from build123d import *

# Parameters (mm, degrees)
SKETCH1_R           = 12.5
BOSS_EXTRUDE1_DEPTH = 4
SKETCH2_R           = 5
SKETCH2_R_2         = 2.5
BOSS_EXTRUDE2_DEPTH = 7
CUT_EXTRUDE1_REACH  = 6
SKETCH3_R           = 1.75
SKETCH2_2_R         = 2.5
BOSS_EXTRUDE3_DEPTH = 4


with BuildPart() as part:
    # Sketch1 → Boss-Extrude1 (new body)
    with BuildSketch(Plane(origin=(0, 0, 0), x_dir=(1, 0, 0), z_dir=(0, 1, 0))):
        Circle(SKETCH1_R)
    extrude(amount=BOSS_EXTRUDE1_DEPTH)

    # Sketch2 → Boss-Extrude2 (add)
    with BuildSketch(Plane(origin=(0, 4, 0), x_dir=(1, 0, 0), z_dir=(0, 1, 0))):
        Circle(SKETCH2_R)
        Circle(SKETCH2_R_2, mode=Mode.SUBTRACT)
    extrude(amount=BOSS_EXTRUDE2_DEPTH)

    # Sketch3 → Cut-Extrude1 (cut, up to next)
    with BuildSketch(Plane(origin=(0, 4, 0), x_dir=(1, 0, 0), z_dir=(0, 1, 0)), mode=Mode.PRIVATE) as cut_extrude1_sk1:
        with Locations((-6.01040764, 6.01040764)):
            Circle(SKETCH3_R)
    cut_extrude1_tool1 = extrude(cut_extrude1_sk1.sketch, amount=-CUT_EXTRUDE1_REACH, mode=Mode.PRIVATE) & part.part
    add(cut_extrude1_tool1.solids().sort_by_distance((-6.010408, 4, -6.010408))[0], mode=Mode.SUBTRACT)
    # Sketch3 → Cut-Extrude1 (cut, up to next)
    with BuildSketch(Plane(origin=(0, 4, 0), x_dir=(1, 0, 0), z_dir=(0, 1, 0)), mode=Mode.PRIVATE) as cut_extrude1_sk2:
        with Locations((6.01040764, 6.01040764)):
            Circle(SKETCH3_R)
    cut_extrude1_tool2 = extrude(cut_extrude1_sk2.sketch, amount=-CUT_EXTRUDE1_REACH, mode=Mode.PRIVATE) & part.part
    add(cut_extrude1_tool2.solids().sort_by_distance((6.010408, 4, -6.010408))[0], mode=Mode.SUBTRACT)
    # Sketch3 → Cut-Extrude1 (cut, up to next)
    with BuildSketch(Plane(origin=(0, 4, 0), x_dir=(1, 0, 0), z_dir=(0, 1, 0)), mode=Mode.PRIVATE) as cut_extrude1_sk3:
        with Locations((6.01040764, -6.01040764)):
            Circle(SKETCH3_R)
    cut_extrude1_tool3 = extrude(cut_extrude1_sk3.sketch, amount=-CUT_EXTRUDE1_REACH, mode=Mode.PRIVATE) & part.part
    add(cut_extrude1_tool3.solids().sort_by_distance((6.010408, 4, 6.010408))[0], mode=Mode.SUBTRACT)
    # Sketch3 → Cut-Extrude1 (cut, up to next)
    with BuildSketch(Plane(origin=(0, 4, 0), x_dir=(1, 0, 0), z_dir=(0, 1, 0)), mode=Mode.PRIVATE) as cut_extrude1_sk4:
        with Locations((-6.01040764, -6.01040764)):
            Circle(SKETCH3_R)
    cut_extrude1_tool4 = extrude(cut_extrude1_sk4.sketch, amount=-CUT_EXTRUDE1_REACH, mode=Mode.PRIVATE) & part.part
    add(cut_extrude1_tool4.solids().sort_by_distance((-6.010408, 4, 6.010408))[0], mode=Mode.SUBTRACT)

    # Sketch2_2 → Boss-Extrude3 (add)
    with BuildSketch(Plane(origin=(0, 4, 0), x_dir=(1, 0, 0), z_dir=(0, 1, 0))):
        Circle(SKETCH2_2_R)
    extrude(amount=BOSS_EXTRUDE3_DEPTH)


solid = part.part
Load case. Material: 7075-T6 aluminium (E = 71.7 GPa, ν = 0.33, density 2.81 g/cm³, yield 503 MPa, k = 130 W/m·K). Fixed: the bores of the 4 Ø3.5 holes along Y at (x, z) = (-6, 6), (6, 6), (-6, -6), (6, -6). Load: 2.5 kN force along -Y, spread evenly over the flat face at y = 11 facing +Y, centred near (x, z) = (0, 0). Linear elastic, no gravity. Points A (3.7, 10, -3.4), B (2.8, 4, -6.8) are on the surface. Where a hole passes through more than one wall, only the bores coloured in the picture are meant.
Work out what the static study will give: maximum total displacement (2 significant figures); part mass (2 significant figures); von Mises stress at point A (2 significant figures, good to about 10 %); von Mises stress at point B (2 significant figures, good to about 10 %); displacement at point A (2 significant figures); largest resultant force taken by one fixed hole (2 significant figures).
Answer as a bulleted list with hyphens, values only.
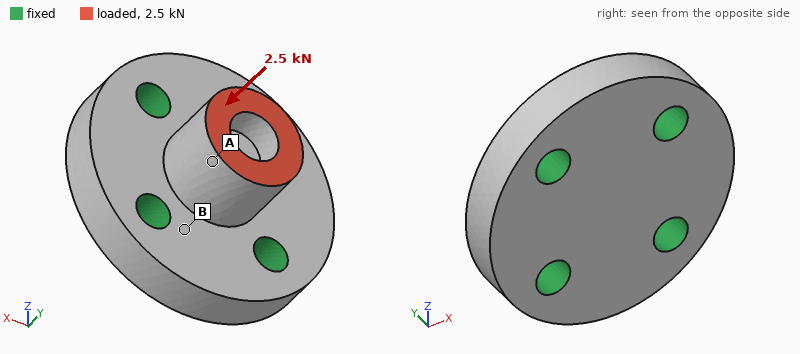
- 8.2 µm
- 6.5 g
- 43 MPa
- 13 MPa
- 7.5 µm
- 650 N
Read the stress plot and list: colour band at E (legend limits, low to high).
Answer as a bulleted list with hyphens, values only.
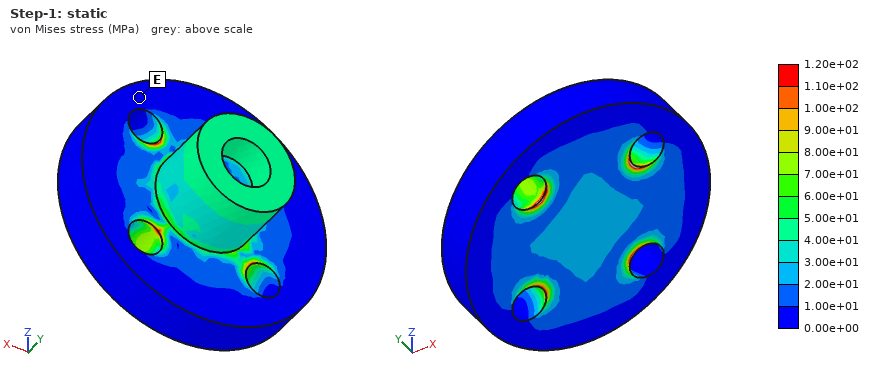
- 0.00e+00 to 1.00e+01 MPa
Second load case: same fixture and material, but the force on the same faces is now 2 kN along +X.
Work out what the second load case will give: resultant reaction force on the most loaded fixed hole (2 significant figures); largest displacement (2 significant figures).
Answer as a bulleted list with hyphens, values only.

- 990 N
- 37 µm
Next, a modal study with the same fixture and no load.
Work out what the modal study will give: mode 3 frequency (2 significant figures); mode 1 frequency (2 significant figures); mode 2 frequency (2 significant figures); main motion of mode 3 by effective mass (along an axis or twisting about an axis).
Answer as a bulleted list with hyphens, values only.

- 73 kHz
- 57 kHz
- 57 kHz
- along Y
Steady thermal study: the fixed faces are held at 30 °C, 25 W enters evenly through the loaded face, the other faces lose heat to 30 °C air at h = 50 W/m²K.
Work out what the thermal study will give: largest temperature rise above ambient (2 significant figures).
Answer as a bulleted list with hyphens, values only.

- 28 K
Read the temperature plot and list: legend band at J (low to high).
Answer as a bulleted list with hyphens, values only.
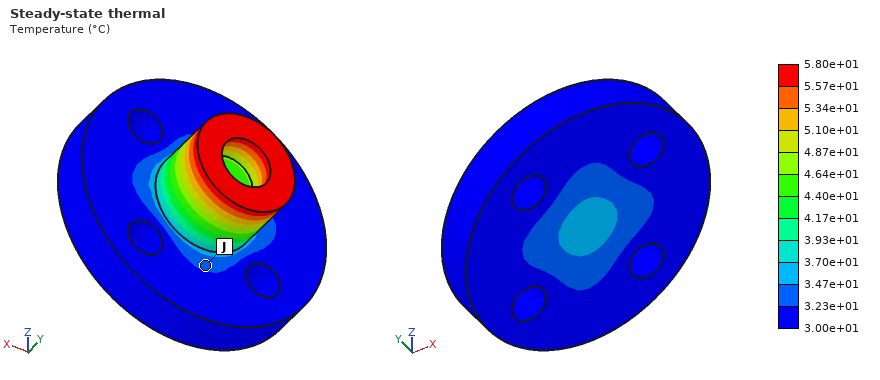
- 3.23e+01 to 3.47e+01 °C
